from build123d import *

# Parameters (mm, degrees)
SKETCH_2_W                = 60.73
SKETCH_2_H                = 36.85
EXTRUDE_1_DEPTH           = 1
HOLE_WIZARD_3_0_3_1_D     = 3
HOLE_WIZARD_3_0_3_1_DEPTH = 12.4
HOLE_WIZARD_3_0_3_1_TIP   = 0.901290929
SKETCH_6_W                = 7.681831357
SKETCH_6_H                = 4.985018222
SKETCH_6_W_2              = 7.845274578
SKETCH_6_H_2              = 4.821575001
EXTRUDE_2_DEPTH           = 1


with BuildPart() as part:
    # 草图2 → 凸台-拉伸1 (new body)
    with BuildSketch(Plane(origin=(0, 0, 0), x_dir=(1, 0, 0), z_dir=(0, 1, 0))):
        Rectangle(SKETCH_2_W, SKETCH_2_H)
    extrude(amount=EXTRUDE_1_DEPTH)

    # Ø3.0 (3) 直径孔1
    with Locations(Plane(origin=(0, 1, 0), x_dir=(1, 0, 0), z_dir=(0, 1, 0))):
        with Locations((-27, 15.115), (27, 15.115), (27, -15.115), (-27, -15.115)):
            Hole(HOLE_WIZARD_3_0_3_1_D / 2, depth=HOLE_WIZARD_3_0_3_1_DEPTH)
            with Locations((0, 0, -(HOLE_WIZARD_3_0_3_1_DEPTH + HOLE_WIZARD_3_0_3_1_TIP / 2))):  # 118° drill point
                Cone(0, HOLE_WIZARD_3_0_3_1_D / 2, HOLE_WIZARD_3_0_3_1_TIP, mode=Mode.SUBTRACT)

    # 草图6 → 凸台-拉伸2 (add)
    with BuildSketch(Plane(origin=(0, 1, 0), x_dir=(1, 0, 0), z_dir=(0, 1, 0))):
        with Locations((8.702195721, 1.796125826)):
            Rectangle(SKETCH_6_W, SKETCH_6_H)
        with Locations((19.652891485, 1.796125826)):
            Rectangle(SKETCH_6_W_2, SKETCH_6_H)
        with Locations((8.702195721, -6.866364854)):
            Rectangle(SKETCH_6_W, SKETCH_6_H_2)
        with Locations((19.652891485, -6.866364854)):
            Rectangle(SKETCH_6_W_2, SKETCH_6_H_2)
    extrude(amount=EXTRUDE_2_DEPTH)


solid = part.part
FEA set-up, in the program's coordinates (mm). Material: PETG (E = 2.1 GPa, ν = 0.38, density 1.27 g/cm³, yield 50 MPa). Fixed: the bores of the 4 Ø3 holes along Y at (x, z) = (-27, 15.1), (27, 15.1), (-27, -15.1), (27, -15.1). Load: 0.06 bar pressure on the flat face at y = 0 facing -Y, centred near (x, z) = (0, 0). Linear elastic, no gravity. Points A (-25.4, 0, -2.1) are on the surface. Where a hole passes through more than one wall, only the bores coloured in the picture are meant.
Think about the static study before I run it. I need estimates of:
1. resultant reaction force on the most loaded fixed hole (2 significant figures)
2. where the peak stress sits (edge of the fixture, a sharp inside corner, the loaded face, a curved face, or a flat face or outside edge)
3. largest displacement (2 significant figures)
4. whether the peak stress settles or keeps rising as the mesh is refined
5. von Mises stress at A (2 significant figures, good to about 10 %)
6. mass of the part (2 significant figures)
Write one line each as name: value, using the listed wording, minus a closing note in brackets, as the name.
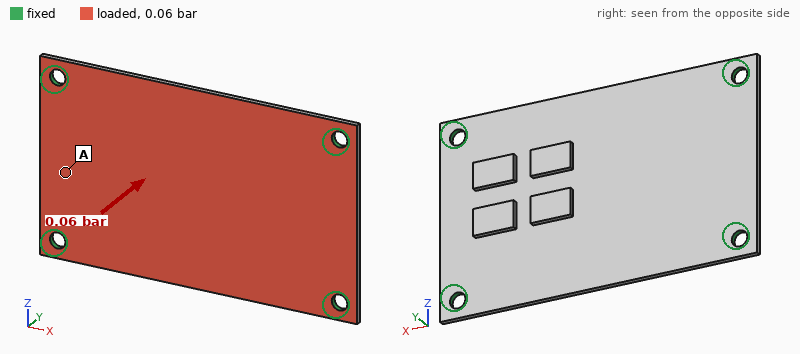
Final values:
resultant reaction force on the most loaded fixed hole: 3.4 N
where the peak stress sits: edge of the fixture
largest displacement: 0.82 mm
whether the peak stress settles or keeps rising as the mesh is refined: keeps rising
von Mises stress at A: 2.0 MPa
mass of the part: 3.0 g
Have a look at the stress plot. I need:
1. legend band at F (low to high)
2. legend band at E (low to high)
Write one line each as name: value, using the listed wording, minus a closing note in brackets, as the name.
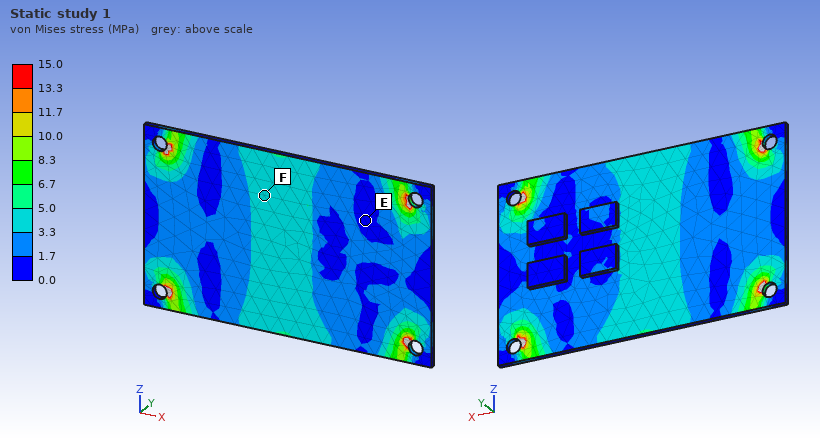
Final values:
legend band at F: 3.3 to 5.0 MPa
legend band at E: 0.0 to 1.7 MPa
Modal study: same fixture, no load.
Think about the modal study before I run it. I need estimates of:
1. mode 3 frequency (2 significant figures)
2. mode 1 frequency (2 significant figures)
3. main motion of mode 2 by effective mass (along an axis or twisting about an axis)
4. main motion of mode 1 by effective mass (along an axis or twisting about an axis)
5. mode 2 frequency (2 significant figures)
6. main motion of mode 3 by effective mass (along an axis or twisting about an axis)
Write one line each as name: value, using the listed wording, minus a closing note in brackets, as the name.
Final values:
mode 3 frequency: 1200 Hz
mode 1 frequency: 430 Hz
main motion of mode 2 by effective mass: twisting about X
main motion of mode 1 by effective mass: along Y
mode 2 frequency: 720 Hz
main motion of mode 3 by effective mass: twisting about Z
